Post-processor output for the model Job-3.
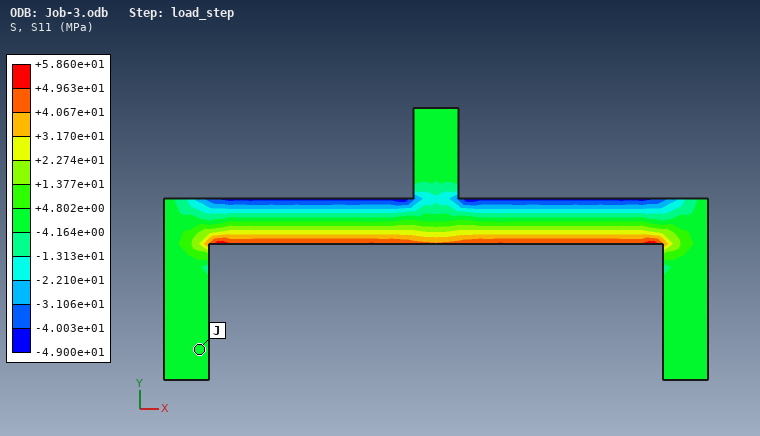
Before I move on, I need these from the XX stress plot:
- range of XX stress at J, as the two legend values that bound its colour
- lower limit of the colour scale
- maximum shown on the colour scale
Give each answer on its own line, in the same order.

-4.164e+00 to +4.802e+00 MPa
-4.900e+01 MPa
+5.860e+01 MPa
